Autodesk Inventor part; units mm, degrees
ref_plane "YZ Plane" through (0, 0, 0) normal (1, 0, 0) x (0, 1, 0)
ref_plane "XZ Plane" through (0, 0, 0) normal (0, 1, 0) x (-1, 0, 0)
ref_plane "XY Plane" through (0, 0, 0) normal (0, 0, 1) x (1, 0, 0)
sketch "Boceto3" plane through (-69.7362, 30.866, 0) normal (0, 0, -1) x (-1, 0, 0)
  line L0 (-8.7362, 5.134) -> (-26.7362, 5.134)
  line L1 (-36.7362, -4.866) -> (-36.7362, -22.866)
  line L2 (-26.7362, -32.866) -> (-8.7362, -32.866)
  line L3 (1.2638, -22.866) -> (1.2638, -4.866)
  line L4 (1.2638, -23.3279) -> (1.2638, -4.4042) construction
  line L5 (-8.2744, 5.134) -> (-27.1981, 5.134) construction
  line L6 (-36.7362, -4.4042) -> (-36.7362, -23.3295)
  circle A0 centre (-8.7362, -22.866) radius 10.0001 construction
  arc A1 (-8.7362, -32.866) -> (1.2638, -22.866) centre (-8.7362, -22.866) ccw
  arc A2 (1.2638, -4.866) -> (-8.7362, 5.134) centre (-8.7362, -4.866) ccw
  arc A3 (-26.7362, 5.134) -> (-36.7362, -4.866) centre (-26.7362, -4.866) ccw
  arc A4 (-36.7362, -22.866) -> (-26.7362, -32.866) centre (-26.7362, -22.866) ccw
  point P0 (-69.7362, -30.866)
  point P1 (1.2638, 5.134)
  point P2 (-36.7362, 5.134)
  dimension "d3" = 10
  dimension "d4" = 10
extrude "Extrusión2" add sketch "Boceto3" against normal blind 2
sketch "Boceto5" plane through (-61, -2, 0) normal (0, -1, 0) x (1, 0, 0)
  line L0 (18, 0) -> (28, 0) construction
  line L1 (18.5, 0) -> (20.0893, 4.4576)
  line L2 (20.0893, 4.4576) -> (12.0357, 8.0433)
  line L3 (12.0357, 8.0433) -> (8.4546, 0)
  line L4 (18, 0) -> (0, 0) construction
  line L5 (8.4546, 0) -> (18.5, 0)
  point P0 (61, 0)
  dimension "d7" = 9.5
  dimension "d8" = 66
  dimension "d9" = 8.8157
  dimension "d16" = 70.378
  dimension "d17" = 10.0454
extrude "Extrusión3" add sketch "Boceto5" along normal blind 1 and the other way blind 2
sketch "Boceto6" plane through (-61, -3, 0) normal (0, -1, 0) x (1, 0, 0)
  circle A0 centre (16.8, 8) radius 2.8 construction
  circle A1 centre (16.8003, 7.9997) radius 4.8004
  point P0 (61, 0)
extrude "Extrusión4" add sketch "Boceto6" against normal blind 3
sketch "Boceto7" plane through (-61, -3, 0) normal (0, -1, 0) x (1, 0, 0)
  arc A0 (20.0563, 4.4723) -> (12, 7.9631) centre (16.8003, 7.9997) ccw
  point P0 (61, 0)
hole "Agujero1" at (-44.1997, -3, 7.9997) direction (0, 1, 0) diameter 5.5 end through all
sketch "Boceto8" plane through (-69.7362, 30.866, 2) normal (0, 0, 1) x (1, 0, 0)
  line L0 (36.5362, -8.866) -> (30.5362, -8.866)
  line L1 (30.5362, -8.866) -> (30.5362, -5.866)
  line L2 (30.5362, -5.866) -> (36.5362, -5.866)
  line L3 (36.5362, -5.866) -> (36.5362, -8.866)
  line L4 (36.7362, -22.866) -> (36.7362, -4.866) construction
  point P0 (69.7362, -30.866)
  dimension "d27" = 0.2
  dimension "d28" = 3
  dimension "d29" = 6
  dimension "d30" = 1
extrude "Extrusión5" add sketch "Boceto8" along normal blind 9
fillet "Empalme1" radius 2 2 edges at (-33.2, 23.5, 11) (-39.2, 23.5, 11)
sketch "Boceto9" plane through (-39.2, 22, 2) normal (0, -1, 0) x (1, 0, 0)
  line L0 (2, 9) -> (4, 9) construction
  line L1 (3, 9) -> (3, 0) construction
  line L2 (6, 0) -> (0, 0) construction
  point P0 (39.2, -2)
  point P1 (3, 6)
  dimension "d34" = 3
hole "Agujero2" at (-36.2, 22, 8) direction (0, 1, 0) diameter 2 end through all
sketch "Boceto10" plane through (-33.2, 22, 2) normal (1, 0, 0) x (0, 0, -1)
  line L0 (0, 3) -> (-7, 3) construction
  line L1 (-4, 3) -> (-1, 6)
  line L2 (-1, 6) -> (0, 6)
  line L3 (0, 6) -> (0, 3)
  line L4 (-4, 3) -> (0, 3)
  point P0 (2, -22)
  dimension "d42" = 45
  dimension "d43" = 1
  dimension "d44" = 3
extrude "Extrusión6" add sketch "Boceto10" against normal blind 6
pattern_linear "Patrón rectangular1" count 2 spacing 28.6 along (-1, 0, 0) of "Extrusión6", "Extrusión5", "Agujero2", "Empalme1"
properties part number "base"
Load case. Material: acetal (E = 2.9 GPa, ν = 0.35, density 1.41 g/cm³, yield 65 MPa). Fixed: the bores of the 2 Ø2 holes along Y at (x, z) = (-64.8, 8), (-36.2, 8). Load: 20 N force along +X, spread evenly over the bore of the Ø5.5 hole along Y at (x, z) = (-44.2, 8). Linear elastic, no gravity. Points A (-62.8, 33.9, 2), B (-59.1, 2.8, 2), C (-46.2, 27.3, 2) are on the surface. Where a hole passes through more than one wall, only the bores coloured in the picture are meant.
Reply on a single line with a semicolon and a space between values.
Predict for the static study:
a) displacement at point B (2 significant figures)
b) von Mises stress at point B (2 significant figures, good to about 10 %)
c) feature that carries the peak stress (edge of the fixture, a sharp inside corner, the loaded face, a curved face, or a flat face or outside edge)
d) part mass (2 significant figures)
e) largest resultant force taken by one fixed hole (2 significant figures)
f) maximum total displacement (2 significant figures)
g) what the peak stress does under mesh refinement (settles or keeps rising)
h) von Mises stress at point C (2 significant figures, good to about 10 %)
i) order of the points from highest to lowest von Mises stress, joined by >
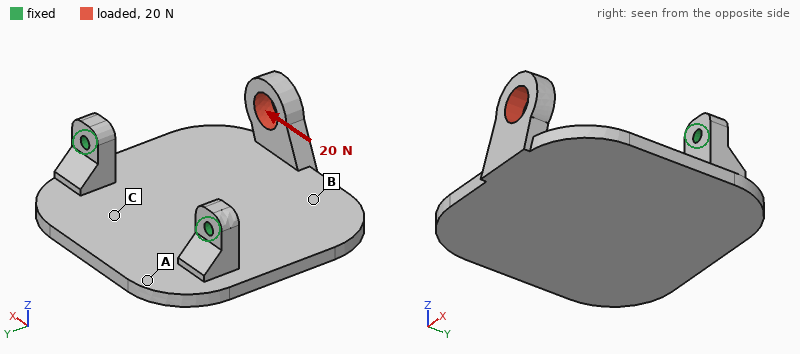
0.23 mm; 4.0 MPa; edge of the fixture; 4.7 g; 19 N; 0.58 mm; keeps rising; 2.2 MPa; B > C > A
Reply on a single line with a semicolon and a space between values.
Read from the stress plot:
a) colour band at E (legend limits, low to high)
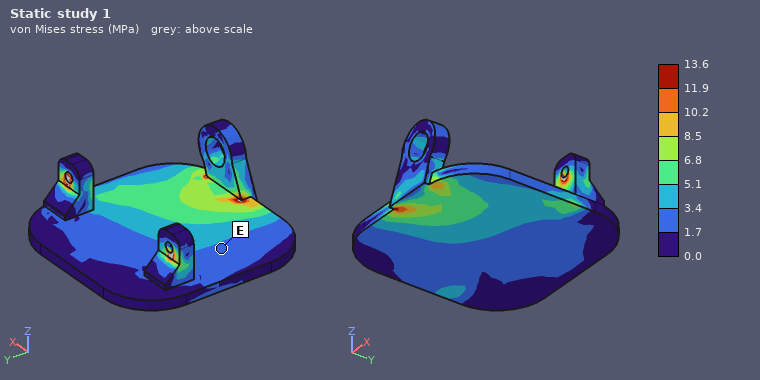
1.7 to 3.4 MPa
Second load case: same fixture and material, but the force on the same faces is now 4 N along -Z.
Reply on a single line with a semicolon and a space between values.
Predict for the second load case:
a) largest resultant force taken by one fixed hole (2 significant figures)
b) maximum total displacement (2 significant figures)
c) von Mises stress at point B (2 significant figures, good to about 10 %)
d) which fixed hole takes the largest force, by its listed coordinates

3.5 N; 0.58 mm; 1.3 MPa; (-36.2, 8)
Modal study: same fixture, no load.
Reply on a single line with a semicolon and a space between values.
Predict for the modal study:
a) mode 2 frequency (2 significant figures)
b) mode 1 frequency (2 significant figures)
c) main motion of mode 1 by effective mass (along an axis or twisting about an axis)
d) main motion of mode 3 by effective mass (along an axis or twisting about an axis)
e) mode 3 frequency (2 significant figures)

1200 Hz; 470 Hz; along Z; along Y; 1800 Hz
